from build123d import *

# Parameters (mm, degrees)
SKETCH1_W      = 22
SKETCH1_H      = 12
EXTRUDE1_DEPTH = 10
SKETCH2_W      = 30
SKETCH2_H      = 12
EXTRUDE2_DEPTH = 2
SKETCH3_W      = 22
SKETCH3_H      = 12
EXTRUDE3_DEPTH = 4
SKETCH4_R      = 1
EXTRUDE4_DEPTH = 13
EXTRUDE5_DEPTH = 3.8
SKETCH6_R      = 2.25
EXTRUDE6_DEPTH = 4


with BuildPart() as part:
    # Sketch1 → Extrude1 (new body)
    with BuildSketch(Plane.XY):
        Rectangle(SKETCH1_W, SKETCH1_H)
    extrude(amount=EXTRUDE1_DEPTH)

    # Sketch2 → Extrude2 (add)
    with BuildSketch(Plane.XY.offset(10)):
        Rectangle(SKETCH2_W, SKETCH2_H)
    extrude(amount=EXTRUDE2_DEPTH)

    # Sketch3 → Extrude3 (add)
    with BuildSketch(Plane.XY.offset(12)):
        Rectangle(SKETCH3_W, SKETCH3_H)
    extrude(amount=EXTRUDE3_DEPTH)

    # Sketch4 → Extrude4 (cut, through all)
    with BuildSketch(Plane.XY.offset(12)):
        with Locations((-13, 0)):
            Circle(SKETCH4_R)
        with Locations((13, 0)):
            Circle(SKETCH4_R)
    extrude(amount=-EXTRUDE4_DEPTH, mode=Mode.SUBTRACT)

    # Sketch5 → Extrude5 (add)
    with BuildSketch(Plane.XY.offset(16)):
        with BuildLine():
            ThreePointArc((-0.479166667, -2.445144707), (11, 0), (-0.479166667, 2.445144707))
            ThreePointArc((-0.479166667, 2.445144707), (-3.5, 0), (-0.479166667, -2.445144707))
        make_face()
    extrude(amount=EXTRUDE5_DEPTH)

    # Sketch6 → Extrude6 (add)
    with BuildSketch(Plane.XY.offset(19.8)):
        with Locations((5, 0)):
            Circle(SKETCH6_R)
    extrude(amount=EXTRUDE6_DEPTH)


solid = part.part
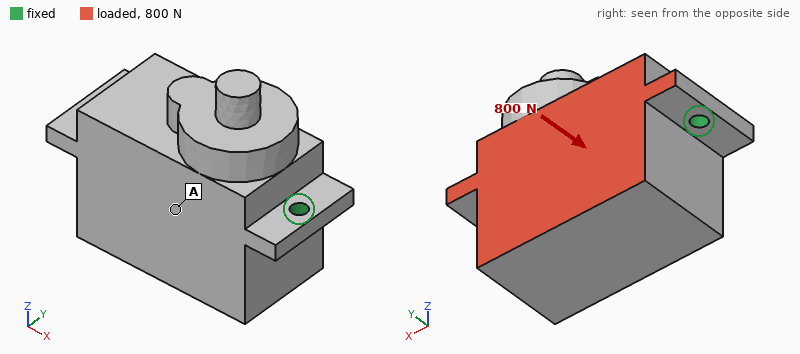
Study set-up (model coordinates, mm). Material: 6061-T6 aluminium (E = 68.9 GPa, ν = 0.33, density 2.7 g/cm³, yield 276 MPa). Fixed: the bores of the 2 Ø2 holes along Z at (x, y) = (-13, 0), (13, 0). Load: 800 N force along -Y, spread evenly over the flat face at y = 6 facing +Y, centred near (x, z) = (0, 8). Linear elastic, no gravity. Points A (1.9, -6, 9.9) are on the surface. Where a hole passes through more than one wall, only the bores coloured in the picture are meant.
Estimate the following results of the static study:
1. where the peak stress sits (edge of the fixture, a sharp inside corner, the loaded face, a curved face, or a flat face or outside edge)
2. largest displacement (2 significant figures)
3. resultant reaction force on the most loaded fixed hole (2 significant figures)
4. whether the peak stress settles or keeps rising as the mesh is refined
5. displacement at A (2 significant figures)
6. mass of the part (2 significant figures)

edge of the fixture
48 µm
400 N
keeps rising
22 µm
13 g
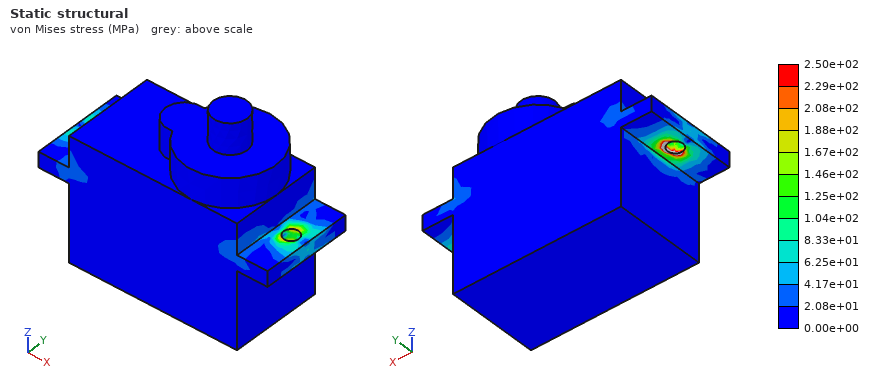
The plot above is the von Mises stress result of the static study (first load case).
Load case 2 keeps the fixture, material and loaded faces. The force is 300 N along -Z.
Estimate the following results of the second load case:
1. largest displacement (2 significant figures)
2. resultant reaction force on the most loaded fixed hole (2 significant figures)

35 µm
150 N
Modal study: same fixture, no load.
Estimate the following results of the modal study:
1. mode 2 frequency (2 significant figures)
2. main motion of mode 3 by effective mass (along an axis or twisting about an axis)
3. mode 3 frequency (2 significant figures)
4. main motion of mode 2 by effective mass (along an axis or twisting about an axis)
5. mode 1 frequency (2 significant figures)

18 kHz
along Y
20 kHz
along Z
5400 Hz
